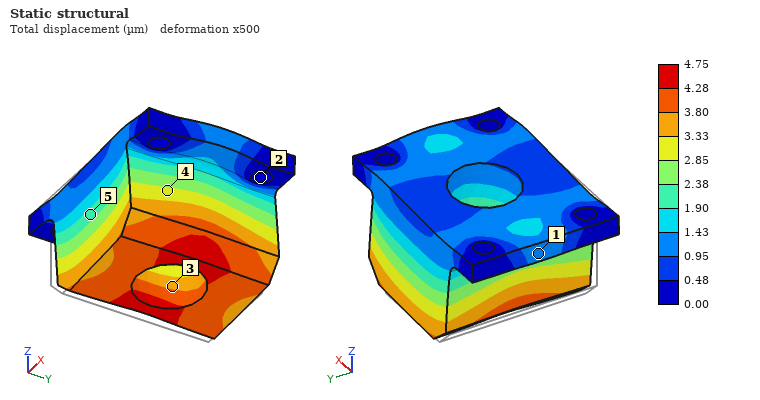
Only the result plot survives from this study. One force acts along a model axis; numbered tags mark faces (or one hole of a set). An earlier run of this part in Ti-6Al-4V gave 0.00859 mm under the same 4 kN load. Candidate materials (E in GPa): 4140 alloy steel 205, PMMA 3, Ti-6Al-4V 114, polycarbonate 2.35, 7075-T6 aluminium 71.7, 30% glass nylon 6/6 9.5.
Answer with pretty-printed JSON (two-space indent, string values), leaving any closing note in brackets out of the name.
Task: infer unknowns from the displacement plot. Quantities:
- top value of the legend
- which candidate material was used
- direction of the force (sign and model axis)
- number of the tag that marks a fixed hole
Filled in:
{
  "top value of the legend": "4.75 µm",
  "which candidate material was used": "4140 alloy steel",
  "direction of the force": "+X",
  "number of the tag that marks a fixed hole": "2"
}
